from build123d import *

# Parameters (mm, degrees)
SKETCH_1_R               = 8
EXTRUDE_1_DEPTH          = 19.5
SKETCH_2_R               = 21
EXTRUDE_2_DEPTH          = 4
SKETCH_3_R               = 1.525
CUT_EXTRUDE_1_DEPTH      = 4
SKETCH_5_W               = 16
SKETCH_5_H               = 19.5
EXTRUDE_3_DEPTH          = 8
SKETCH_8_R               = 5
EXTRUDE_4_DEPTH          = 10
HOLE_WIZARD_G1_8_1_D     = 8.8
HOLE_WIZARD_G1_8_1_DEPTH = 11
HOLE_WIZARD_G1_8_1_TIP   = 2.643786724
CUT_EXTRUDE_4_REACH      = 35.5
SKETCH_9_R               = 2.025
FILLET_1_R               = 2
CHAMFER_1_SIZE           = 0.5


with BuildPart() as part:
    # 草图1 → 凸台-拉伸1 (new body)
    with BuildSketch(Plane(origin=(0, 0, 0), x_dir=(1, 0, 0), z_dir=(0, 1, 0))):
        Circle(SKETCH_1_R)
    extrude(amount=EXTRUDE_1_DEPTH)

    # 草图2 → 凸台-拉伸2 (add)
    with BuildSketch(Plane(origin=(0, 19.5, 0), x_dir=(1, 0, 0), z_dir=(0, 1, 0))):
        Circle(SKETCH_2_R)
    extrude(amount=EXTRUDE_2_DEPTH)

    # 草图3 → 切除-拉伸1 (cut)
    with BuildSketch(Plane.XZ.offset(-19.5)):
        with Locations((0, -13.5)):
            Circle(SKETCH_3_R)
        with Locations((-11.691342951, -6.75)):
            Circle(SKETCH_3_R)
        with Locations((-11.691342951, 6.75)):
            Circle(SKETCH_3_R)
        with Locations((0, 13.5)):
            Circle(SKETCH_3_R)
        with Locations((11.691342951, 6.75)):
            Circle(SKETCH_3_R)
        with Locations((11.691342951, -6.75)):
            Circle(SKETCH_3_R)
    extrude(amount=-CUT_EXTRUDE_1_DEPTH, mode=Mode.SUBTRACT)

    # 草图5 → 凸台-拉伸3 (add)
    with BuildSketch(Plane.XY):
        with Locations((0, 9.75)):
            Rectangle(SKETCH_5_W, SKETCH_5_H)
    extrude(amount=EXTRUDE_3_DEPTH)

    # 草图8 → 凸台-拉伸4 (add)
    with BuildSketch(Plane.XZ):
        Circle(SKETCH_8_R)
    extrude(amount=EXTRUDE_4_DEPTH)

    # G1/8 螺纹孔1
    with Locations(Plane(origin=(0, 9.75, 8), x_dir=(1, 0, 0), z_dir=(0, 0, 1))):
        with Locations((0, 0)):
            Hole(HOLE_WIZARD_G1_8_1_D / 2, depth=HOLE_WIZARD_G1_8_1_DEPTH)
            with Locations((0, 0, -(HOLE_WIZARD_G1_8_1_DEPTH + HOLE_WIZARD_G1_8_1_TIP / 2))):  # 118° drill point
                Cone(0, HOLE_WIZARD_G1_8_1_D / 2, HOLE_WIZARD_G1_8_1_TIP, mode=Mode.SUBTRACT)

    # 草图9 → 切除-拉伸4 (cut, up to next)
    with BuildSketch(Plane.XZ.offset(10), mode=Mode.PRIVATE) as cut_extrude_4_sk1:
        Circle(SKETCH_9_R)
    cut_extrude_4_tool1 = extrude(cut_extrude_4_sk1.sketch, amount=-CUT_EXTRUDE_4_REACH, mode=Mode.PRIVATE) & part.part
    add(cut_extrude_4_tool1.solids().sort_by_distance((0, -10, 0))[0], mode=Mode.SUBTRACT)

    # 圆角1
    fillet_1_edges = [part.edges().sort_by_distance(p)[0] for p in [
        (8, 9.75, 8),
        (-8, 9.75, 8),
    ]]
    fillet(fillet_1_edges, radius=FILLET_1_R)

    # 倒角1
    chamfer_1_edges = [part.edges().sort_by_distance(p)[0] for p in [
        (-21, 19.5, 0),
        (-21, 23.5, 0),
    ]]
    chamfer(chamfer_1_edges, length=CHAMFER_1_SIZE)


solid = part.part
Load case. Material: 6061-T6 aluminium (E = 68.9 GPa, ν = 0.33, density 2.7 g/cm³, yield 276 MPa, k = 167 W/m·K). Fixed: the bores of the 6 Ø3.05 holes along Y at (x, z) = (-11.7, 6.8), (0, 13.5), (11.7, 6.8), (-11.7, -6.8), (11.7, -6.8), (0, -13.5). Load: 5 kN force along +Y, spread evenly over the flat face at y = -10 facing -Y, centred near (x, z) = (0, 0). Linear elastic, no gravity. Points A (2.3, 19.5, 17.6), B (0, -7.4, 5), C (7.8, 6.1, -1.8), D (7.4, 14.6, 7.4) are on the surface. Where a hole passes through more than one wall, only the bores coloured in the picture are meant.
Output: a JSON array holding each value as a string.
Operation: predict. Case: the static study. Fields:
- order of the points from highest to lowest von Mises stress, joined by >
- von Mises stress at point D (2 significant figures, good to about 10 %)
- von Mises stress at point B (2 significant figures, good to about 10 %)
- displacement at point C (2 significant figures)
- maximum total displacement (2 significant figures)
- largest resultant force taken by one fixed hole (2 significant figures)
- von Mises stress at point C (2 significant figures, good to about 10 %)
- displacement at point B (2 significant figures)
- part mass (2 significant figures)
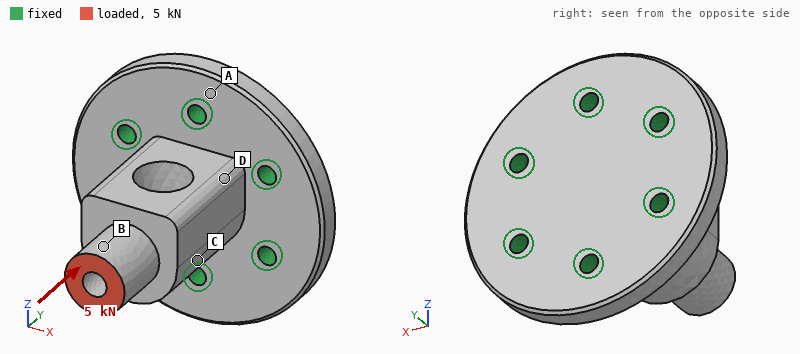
["B > D > C > A", "54 MPa", "75 MPa", "18 µm", "35 µm", "990 N", "27 MPa", "32 µm", "26 g"]
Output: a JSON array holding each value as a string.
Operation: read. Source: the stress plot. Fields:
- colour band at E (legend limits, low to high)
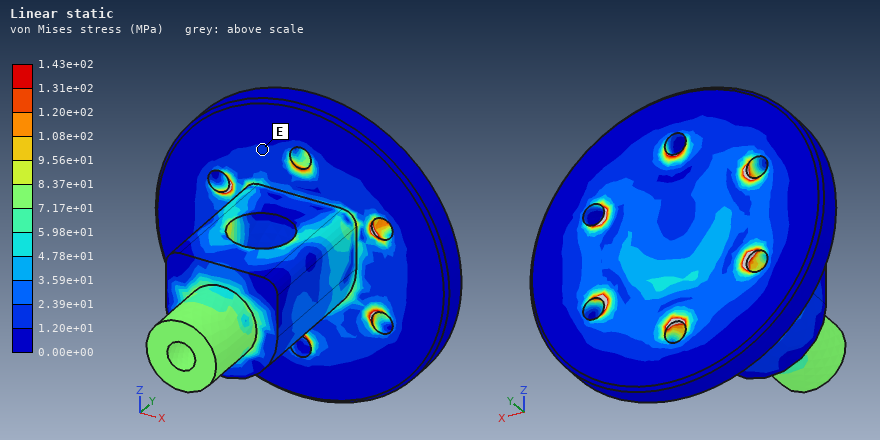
["1.20e+01 to 2.39e+01 MPa"]
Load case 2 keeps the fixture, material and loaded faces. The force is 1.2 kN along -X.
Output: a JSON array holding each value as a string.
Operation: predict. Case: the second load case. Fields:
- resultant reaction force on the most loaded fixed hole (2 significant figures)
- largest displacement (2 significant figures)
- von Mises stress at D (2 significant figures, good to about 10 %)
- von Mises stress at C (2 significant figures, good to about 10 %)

["1.2 kN", "0.12 mm", "74 MPa", "34 MPa"]
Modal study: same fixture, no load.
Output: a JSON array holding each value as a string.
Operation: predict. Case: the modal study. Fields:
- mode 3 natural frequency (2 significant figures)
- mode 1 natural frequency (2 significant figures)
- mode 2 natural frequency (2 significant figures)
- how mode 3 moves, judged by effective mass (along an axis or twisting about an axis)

["25 kHz", "11 kHz", "11 kHz", "along Y"]
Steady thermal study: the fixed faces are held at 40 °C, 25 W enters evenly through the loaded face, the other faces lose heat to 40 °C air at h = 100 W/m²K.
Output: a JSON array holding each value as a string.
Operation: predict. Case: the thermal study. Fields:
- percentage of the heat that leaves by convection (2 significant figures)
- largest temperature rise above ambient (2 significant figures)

["15 %", "44 K"]
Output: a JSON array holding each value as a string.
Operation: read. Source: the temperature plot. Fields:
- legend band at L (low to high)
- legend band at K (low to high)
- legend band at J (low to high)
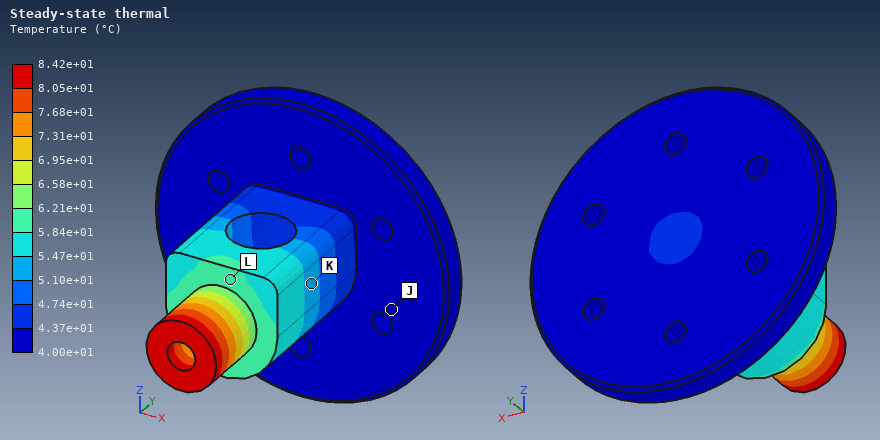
["5.84e+01 to 6.21e+01 °C", "5.10e+01 to 5.47e+01 °C", "4.00e+01 to 4.37e+01 °C"]
